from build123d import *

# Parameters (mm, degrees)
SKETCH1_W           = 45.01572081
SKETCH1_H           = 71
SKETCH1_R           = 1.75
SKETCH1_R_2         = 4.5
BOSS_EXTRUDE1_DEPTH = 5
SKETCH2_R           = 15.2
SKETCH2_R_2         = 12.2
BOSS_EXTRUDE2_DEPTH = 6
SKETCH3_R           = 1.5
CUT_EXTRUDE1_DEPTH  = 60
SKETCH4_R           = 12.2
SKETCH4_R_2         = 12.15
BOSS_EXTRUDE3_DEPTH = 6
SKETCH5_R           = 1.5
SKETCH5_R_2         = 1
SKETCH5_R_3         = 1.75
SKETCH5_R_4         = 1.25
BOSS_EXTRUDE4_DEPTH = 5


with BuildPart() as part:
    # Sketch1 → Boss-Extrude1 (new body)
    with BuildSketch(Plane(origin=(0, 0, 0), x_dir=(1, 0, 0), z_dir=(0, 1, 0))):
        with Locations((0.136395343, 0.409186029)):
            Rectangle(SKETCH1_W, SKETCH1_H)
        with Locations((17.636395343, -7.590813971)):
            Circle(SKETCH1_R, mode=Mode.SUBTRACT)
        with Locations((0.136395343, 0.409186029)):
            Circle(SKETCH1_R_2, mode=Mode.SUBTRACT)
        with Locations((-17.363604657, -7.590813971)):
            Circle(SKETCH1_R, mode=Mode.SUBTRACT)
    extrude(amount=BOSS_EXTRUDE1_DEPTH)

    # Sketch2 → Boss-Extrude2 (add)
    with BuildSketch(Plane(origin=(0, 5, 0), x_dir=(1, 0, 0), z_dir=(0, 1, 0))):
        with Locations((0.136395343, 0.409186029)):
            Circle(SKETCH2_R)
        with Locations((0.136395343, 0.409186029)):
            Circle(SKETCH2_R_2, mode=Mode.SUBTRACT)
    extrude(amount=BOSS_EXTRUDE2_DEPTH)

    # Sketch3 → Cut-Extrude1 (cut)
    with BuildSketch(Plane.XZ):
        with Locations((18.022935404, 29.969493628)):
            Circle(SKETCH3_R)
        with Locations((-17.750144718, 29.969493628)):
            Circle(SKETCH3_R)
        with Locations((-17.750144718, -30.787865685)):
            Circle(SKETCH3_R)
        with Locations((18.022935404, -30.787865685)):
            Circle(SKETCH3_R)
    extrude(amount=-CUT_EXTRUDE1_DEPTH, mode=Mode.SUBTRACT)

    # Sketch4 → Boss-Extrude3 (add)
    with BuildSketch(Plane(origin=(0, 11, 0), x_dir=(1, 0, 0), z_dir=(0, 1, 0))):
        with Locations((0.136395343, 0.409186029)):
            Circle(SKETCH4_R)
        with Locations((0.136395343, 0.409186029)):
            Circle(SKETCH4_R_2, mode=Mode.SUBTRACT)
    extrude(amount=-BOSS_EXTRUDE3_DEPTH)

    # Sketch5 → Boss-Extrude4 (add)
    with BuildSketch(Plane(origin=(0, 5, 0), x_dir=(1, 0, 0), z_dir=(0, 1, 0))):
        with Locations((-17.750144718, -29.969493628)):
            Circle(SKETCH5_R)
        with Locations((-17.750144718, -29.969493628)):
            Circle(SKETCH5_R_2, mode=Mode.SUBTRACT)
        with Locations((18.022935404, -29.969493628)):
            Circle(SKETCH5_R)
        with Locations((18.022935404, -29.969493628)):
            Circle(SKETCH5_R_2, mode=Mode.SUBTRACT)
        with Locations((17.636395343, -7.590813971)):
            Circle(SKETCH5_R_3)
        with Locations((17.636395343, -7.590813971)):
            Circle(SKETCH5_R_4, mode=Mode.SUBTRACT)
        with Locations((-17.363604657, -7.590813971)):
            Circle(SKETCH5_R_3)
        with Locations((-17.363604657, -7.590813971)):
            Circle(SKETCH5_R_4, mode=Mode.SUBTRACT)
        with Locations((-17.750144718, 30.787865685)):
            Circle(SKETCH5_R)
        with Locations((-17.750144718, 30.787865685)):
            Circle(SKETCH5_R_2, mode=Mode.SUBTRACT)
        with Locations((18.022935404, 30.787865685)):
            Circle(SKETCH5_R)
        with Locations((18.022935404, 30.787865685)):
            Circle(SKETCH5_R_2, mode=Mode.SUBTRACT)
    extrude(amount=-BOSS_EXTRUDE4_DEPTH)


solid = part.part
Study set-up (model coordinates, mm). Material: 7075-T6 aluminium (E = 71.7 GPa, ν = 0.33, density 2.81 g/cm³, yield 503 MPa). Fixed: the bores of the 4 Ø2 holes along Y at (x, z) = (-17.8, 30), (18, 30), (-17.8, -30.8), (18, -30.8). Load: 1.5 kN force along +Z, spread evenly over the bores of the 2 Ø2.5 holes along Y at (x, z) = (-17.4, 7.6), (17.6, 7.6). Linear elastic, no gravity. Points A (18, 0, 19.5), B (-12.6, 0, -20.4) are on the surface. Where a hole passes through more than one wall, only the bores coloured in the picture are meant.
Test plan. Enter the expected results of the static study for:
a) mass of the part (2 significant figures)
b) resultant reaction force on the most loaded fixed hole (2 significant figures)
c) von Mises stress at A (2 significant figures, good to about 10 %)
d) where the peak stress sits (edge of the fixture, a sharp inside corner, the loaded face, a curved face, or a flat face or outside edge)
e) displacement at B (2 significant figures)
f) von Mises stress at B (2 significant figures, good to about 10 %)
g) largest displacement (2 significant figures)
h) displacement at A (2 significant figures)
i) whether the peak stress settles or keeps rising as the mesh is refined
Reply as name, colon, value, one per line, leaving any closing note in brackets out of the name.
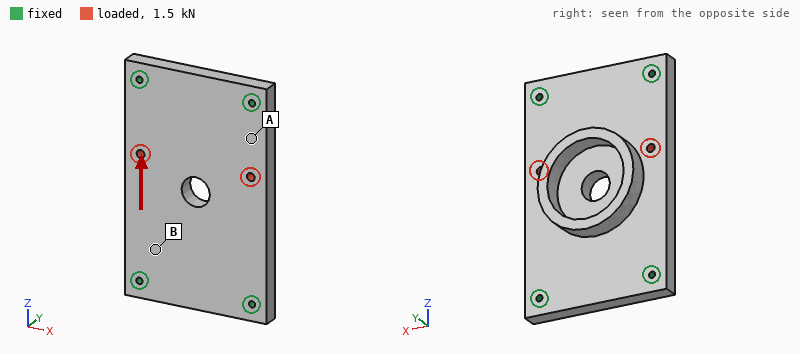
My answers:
mass of the part: 48 g
resultant reaction force on the most loaded fixed hole: 450 N
von Mises stress at A: 7.6 MPa
where the peak stress sits: edge of the fixture
displacement at B: 1.0 µm
von Mises stress at B: 3.1 MPa
largest displacement: 3.1 µm
displacement at A: 1.4 µm
whether the peak stress settles or keeps rising as the mesh is refined: keeps rising
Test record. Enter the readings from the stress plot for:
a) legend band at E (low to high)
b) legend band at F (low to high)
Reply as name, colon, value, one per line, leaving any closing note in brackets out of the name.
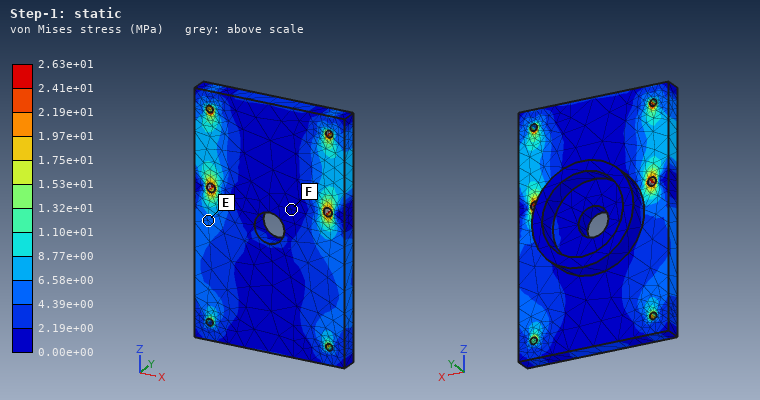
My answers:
legend band at E: 4.39e+00 to 6.58e+00 MPa
legend band at F: 0.00e+00 to 2.19e+00 MPa
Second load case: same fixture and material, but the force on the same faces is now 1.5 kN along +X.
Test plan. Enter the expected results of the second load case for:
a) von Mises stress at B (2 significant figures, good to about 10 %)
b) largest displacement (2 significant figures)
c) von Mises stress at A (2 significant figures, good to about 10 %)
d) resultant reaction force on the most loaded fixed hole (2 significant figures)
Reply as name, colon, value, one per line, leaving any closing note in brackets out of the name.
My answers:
von Mises stress at B: 4.4 MPa
largest displacement: 6.7 µm
von Mises stress at A: 5.0 MPa
resultant reaction force on the most loaded fixed hole: 570 N
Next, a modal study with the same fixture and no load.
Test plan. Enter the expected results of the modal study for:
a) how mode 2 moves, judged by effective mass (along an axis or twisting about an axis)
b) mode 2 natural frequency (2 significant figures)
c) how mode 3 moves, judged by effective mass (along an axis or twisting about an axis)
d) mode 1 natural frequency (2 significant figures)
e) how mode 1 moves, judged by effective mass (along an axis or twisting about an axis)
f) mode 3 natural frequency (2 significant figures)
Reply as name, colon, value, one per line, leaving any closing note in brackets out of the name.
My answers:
how mode 2 moves, judged by effective mass: twisting about Z
mode 2 natural frequency: 8100 Hz
how mode 3 moves, judged by effective mass: twisting about X
mode 1 natural frequency: 5400 Hz
how mode 1 moves, judged by effective mass: along Y
mode 3 natural frequency: 13 kHz
